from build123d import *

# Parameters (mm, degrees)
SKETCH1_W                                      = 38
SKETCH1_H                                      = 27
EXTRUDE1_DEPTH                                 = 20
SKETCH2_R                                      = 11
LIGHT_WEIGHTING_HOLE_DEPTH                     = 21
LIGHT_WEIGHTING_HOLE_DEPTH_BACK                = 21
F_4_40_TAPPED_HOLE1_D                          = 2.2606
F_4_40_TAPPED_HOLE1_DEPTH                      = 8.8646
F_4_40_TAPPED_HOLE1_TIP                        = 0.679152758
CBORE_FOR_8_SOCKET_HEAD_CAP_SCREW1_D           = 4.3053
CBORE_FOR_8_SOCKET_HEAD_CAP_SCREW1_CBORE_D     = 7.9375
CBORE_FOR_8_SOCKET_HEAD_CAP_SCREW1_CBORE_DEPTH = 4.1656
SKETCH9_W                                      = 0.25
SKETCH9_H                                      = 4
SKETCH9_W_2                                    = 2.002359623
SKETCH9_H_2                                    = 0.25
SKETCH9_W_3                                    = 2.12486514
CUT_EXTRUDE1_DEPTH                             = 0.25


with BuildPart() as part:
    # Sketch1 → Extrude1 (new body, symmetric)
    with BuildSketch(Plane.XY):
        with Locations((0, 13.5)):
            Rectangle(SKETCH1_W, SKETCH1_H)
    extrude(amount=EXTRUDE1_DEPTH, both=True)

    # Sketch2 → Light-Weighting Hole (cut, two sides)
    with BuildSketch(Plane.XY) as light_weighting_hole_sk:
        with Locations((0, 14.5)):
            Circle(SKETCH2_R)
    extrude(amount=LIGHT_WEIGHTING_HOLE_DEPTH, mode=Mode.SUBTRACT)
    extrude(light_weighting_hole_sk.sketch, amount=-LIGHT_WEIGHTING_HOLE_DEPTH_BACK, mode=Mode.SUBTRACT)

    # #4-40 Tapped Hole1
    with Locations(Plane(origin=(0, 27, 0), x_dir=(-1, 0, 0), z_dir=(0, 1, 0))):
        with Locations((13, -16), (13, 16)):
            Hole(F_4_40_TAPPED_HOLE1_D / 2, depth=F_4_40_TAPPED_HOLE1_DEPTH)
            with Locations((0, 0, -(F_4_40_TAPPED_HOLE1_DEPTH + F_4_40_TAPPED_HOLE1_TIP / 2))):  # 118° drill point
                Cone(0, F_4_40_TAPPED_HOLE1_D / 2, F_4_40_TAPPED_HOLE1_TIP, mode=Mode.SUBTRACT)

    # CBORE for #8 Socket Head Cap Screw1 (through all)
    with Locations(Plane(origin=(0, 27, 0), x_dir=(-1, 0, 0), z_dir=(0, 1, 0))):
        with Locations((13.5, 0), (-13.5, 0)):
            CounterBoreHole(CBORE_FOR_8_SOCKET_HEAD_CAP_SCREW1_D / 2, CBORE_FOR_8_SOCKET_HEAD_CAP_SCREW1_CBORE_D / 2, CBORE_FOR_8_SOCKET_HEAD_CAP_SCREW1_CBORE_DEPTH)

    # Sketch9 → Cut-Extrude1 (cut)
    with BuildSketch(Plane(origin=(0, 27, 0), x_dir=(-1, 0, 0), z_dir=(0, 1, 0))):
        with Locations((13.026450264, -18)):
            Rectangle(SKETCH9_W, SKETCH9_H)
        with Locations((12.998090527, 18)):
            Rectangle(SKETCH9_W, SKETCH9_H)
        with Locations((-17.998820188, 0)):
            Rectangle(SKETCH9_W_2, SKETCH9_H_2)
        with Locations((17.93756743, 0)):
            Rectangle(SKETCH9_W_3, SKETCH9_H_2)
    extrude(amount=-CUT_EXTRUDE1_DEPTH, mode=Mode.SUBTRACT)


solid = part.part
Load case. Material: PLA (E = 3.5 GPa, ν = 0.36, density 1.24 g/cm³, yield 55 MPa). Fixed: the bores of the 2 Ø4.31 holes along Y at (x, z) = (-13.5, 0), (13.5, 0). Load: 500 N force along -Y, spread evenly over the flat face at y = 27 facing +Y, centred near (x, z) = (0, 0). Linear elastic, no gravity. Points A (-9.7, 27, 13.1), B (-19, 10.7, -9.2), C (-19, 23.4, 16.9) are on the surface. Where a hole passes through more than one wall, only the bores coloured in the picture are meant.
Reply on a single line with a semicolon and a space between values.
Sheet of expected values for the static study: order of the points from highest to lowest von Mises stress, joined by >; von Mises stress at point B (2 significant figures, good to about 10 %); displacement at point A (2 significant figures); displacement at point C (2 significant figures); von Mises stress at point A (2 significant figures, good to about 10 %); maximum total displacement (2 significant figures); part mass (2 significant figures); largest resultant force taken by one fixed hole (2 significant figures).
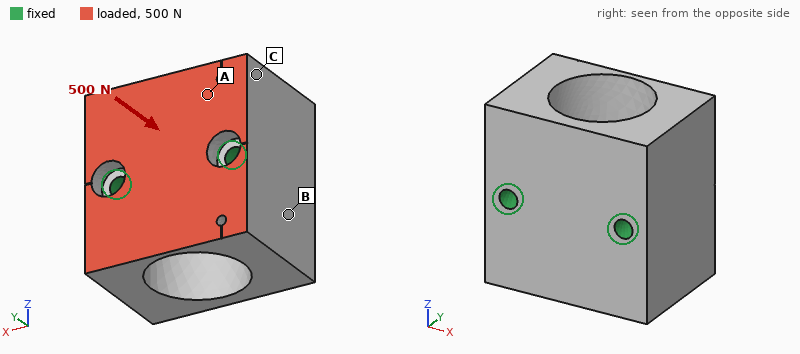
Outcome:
A > B > C; 0.88 MPa; 11 µm; 5.9 µm; 1.4 MPa; 33 µm; 31 g; 260 N
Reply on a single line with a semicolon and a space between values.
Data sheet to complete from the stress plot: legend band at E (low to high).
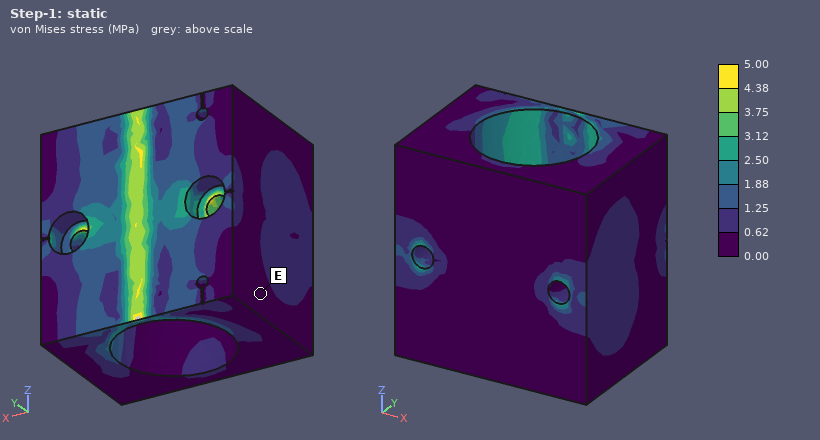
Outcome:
0.00 to 0.62 MPa
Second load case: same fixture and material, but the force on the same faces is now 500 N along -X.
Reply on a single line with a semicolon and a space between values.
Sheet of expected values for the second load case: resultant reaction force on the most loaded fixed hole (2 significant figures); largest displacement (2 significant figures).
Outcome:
260 N; 33 µm
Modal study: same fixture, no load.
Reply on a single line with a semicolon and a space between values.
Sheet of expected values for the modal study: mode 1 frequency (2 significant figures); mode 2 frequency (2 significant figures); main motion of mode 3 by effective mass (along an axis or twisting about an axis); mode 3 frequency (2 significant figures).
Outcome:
7300 Hz; 7500 Hz; along X; 7800 Hz
